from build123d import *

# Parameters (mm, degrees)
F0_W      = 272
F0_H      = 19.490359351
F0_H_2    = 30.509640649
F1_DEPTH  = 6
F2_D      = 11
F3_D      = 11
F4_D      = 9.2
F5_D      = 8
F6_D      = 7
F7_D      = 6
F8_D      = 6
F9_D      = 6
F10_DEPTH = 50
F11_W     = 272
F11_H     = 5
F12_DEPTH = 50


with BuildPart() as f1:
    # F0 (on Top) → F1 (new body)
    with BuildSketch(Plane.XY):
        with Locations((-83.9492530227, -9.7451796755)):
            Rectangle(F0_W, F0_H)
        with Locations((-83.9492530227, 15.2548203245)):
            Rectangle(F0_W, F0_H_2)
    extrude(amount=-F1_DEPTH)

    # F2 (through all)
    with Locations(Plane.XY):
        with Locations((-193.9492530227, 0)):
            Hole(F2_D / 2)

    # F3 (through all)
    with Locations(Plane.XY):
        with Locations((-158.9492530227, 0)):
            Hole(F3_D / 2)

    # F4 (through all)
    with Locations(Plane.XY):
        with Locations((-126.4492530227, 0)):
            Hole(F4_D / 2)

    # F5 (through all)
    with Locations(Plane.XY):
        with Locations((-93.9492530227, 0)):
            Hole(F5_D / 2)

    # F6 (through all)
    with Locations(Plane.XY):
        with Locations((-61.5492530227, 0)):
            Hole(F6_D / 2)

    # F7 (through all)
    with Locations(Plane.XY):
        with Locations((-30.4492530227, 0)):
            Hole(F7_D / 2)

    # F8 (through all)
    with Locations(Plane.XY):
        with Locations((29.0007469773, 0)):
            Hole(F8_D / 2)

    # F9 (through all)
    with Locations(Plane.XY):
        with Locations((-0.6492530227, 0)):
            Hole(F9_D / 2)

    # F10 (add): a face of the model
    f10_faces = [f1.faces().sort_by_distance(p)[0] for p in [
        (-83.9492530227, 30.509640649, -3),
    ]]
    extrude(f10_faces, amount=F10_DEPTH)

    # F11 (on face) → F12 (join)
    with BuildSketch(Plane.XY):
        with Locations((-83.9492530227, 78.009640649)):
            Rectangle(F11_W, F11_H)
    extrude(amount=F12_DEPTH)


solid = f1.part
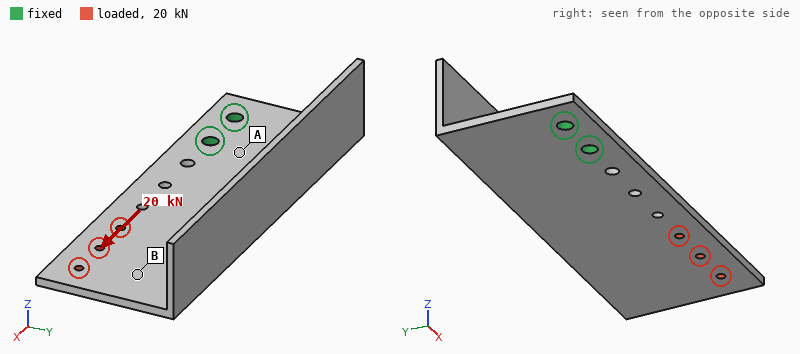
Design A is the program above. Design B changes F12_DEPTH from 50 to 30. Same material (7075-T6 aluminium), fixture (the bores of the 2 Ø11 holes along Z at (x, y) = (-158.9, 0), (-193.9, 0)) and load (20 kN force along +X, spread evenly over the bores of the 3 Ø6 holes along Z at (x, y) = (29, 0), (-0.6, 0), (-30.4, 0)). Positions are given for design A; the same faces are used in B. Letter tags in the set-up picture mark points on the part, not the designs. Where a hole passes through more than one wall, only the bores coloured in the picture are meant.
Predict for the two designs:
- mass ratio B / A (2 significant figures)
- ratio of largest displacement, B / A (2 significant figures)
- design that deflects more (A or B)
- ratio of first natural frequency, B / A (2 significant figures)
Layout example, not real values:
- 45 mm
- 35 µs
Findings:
- 0.88
- 1.1
- B
- 1.1
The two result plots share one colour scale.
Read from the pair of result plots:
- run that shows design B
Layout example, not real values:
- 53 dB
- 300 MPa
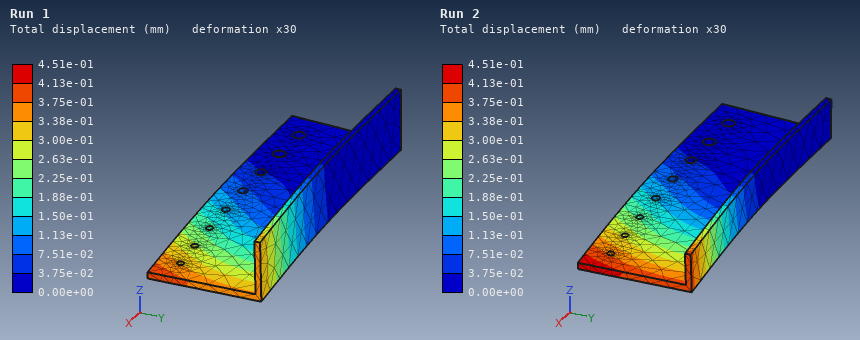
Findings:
- Run 2
